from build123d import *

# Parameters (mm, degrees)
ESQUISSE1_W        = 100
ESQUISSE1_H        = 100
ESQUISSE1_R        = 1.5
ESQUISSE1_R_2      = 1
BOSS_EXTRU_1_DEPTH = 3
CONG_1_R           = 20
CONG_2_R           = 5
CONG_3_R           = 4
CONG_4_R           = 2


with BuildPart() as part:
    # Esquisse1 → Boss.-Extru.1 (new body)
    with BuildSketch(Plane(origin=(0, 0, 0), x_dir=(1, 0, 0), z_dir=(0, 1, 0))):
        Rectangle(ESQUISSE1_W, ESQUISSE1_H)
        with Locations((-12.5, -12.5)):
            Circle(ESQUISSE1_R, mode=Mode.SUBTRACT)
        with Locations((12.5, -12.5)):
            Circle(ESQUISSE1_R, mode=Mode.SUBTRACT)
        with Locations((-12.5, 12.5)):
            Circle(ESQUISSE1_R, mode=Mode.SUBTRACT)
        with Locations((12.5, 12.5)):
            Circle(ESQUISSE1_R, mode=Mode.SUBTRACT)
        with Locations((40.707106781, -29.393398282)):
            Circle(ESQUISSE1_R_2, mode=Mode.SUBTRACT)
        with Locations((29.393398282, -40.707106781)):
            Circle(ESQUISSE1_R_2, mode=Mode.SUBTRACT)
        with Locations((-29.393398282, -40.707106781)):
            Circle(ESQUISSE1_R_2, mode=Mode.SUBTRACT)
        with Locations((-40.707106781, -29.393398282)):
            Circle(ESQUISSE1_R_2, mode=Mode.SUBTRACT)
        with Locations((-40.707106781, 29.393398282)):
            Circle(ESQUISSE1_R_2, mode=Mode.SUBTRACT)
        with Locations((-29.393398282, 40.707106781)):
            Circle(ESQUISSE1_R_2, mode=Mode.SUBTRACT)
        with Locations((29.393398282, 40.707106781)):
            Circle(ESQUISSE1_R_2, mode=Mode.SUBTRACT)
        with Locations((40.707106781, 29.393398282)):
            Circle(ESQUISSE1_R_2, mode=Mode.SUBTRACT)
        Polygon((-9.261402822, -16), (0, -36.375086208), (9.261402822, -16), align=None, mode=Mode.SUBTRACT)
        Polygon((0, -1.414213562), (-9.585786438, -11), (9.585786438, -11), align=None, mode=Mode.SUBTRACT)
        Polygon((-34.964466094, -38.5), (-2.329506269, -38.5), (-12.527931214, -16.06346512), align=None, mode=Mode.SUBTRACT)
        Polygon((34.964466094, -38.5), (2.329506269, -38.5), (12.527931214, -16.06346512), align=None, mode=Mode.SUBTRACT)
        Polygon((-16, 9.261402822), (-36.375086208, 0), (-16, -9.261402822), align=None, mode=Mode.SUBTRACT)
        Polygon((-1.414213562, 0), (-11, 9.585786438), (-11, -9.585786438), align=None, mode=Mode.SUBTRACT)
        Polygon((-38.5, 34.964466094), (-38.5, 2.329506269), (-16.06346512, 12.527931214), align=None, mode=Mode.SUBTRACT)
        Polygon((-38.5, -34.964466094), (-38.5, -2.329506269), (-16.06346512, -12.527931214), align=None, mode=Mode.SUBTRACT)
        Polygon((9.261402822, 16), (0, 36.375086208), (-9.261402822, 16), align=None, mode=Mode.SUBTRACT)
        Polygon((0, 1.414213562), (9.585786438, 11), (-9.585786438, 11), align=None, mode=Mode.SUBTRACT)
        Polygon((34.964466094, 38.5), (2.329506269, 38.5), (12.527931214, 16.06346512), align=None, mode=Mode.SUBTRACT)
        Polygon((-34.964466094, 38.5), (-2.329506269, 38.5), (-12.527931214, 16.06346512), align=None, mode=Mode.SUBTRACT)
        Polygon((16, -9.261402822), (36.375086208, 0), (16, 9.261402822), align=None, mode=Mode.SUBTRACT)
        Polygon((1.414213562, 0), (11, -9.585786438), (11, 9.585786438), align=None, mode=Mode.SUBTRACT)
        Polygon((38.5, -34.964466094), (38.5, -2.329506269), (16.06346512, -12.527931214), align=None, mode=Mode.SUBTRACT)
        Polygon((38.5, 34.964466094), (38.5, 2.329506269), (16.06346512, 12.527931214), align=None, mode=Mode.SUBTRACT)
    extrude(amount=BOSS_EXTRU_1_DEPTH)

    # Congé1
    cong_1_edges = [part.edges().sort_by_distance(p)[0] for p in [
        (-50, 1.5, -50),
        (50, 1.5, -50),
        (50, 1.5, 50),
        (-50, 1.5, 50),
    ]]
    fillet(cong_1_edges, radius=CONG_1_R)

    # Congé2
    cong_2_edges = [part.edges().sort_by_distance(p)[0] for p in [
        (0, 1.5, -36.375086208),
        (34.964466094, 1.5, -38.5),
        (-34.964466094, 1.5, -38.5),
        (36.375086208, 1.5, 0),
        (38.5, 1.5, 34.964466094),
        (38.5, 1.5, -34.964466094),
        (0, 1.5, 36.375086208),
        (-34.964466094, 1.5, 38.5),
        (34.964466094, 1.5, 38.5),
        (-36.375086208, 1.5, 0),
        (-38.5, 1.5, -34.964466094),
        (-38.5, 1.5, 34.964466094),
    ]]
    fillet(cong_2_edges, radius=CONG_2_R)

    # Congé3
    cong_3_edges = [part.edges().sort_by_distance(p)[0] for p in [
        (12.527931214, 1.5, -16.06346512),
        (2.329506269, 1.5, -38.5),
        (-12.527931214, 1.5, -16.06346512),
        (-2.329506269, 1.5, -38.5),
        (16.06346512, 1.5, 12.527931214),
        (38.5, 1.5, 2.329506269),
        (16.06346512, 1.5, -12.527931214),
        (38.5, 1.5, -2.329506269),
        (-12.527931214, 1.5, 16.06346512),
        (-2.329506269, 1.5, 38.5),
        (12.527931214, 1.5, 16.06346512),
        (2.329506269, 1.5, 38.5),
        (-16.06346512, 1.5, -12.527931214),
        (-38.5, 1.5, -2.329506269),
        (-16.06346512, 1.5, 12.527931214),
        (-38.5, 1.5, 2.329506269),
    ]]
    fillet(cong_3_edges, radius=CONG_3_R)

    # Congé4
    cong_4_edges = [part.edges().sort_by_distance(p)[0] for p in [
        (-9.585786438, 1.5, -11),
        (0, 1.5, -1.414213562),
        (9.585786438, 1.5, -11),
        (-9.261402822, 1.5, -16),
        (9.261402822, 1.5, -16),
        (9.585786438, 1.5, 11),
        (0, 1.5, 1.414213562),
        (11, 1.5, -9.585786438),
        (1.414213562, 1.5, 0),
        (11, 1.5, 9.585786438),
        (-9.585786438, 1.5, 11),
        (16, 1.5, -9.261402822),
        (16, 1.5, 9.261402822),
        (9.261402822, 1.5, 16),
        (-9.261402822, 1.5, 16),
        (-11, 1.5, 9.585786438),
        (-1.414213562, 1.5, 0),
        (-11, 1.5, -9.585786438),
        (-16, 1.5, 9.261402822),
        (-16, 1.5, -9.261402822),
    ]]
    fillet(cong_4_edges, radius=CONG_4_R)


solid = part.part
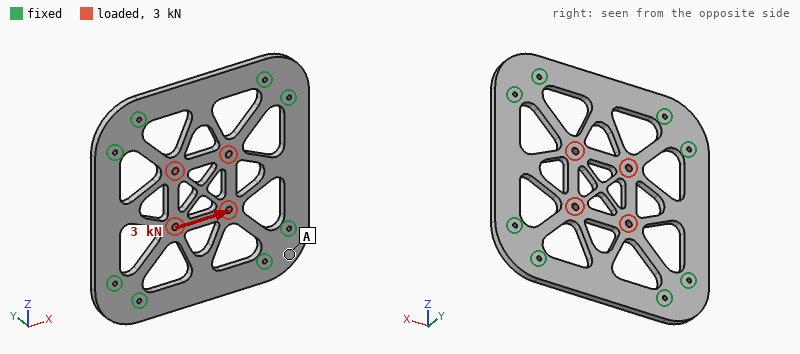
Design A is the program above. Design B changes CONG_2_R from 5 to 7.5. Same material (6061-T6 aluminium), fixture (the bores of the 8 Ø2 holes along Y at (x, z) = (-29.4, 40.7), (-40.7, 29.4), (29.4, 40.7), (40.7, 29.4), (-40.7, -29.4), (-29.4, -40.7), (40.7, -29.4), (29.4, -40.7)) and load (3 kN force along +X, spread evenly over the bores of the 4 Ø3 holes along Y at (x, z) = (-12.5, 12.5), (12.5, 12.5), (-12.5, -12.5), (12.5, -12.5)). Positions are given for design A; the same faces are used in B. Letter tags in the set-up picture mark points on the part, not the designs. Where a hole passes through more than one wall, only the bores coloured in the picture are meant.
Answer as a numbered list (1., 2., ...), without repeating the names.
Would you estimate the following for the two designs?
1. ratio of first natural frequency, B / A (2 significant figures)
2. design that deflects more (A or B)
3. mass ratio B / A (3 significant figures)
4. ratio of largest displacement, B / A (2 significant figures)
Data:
1. 1.1
2. A
3. 1.07
4. 0.84
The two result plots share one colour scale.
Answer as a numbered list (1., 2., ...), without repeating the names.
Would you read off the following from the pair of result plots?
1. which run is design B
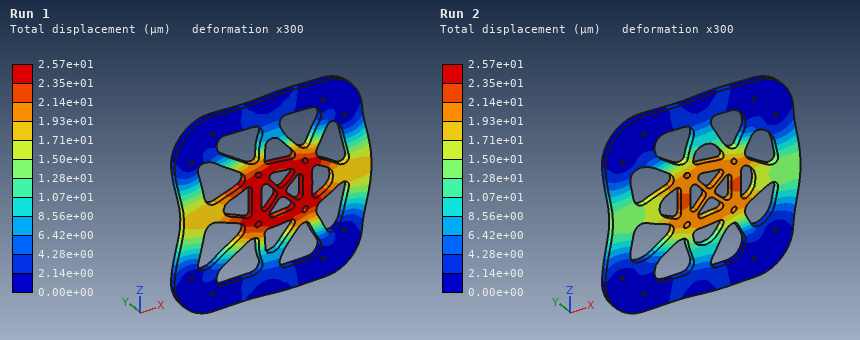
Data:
1. Run 2
